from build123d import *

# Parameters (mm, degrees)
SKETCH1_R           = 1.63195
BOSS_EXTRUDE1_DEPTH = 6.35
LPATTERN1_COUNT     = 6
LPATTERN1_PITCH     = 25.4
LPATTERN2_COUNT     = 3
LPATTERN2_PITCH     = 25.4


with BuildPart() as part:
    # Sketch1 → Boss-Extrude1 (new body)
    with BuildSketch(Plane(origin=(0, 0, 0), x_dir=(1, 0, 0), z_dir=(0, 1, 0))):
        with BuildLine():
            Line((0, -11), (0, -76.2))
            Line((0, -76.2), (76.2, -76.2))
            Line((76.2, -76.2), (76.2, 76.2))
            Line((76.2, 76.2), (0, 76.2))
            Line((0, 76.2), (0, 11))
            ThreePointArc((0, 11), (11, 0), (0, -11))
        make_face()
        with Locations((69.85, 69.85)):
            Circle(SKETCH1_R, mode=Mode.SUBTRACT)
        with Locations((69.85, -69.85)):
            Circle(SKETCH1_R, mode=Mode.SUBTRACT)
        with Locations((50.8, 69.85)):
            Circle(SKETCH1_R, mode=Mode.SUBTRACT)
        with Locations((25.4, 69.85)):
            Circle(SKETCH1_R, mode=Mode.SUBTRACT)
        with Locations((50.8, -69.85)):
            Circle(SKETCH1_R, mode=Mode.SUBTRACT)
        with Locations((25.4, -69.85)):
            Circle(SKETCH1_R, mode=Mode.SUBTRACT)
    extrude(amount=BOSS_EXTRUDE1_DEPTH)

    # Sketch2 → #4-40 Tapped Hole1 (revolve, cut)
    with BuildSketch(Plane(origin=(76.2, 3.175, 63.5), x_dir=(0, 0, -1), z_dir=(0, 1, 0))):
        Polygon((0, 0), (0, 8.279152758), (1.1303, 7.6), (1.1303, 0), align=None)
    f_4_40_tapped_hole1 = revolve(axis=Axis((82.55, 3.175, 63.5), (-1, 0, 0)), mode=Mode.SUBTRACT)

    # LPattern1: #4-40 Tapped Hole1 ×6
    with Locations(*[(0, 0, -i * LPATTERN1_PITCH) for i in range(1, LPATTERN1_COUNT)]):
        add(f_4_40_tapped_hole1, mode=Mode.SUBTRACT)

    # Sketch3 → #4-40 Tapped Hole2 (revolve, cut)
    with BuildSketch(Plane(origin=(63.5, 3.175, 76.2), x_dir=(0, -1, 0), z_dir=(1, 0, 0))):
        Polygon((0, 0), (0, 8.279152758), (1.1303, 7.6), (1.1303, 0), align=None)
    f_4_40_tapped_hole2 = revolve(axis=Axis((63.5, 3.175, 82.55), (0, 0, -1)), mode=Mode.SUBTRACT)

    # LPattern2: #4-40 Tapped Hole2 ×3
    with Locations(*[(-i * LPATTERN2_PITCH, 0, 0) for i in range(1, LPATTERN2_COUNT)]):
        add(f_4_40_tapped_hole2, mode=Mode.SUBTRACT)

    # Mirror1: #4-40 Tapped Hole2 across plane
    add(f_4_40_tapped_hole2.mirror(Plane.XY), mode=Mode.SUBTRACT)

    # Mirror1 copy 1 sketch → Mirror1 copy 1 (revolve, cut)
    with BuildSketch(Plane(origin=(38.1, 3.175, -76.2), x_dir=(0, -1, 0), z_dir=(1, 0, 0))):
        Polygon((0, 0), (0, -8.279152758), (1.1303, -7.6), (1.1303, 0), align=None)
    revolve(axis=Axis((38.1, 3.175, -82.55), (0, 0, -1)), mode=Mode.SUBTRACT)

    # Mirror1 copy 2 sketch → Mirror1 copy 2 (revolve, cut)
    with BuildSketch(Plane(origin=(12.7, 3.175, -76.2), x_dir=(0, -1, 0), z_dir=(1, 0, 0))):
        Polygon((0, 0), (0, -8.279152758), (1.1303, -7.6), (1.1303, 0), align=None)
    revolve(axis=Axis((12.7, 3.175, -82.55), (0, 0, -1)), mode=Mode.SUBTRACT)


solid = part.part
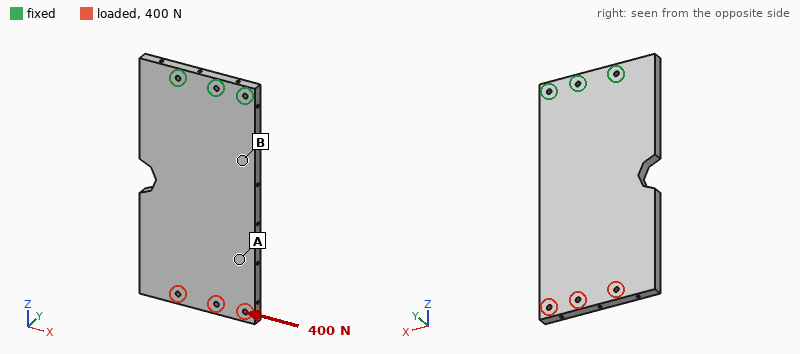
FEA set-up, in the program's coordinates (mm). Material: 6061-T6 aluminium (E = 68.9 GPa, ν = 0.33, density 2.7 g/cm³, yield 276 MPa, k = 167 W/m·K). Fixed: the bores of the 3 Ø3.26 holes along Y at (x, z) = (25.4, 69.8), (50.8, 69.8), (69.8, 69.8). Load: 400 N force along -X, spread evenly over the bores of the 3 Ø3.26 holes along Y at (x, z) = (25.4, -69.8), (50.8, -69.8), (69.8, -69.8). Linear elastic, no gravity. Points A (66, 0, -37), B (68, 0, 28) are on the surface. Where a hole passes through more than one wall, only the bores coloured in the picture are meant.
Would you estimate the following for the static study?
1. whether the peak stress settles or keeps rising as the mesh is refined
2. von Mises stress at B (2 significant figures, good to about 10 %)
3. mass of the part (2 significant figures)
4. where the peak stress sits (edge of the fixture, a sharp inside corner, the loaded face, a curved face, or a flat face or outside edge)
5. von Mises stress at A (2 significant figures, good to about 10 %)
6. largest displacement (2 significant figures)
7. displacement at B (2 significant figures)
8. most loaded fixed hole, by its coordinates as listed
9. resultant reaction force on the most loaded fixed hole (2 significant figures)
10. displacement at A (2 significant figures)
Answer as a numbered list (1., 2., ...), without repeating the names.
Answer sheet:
1. keeps rising
2. 5.9 MPa
3. 190 g
4. edge of the fixture
5. 2.0 MPa
6. 52 µm
7. 11 µm
8. (25.4, 69.8)
9. 1.3 kN
10. 33 µm
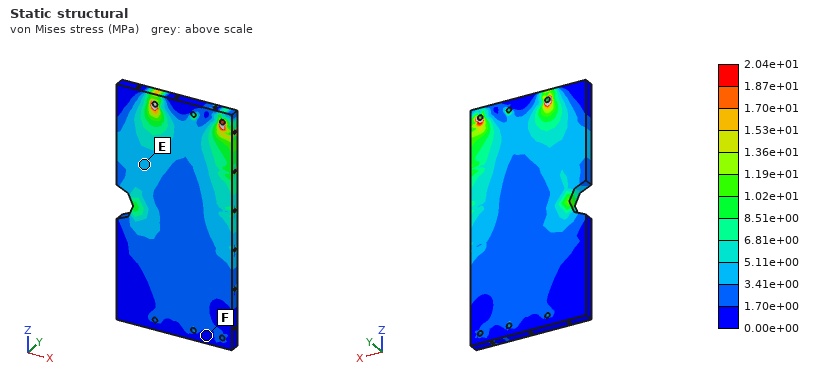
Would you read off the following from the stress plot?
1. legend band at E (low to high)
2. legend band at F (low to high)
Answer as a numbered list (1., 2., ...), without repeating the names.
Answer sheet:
1. 3.41e+00 to 5.11e+00 MPa
2. 0.00e+00 to 1.70e+00 MPa
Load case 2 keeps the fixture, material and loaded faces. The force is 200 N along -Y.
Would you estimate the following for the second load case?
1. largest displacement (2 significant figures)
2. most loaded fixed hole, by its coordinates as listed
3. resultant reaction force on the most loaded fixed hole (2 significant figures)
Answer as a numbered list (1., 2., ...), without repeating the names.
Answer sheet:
1. 1.9 mm
2. (50.8, 69.8)
3. 250 N
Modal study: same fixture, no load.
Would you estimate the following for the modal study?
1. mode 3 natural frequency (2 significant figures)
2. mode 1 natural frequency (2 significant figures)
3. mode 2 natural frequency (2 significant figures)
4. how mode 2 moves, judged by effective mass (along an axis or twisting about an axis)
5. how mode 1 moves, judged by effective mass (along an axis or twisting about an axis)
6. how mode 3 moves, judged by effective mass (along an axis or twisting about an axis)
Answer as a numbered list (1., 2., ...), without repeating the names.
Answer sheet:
1. 1400 Hz
2. 230 Hz
3. 940 Hz
4. twisting about Z
5. along Y
6. along Y
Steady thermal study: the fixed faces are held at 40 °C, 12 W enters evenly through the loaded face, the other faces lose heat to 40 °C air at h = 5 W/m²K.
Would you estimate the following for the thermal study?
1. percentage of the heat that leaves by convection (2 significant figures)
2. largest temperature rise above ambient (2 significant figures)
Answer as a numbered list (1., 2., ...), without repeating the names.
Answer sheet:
1. 12 %
2. 23 K
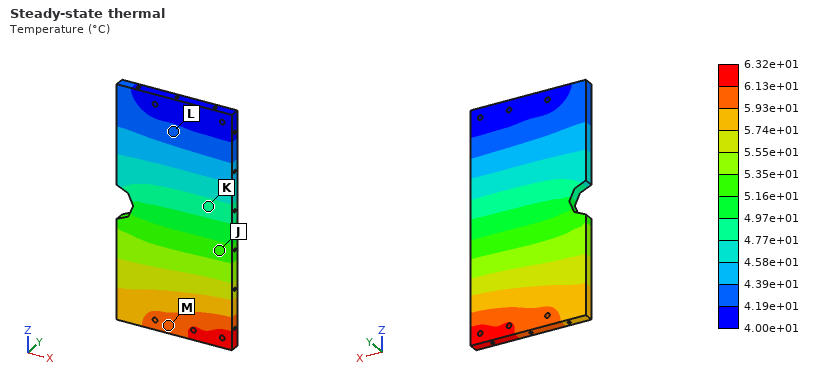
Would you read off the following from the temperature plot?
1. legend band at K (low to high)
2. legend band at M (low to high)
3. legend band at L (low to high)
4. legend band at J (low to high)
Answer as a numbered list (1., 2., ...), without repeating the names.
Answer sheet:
1. 4.77e+01 to 4.97e+01 °C
2. 5.93e+01 to 6.13e+01 °C
3. 4.19e+01 to 4.39e+01 °C
4. 5.16e+01 to 5.35e+01 °C
